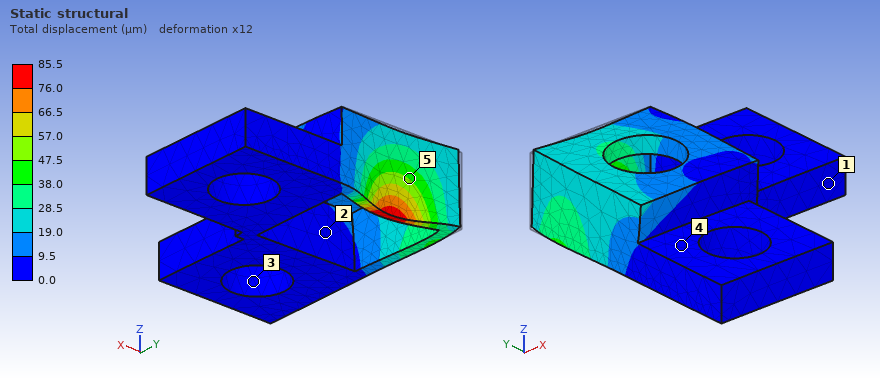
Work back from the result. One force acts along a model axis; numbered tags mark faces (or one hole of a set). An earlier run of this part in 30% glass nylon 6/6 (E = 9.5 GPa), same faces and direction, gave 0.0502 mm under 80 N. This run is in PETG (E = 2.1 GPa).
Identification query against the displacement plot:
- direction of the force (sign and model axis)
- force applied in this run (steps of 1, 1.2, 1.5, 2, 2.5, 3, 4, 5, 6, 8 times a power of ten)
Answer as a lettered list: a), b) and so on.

a) -Y
b) 30 N
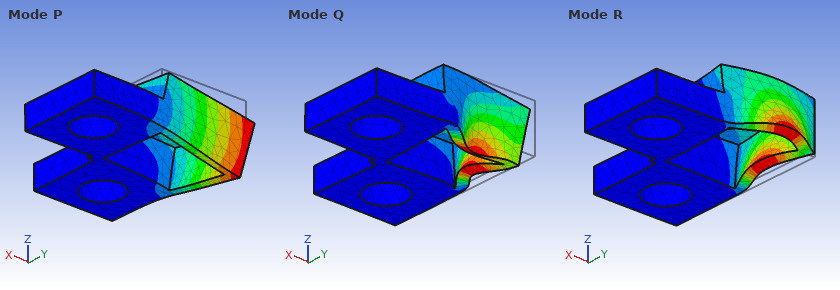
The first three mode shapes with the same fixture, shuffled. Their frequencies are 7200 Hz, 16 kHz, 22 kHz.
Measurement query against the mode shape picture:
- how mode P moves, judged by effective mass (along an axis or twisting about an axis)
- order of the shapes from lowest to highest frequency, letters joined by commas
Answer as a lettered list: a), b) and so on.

a) along Z
b) P, R, Q
